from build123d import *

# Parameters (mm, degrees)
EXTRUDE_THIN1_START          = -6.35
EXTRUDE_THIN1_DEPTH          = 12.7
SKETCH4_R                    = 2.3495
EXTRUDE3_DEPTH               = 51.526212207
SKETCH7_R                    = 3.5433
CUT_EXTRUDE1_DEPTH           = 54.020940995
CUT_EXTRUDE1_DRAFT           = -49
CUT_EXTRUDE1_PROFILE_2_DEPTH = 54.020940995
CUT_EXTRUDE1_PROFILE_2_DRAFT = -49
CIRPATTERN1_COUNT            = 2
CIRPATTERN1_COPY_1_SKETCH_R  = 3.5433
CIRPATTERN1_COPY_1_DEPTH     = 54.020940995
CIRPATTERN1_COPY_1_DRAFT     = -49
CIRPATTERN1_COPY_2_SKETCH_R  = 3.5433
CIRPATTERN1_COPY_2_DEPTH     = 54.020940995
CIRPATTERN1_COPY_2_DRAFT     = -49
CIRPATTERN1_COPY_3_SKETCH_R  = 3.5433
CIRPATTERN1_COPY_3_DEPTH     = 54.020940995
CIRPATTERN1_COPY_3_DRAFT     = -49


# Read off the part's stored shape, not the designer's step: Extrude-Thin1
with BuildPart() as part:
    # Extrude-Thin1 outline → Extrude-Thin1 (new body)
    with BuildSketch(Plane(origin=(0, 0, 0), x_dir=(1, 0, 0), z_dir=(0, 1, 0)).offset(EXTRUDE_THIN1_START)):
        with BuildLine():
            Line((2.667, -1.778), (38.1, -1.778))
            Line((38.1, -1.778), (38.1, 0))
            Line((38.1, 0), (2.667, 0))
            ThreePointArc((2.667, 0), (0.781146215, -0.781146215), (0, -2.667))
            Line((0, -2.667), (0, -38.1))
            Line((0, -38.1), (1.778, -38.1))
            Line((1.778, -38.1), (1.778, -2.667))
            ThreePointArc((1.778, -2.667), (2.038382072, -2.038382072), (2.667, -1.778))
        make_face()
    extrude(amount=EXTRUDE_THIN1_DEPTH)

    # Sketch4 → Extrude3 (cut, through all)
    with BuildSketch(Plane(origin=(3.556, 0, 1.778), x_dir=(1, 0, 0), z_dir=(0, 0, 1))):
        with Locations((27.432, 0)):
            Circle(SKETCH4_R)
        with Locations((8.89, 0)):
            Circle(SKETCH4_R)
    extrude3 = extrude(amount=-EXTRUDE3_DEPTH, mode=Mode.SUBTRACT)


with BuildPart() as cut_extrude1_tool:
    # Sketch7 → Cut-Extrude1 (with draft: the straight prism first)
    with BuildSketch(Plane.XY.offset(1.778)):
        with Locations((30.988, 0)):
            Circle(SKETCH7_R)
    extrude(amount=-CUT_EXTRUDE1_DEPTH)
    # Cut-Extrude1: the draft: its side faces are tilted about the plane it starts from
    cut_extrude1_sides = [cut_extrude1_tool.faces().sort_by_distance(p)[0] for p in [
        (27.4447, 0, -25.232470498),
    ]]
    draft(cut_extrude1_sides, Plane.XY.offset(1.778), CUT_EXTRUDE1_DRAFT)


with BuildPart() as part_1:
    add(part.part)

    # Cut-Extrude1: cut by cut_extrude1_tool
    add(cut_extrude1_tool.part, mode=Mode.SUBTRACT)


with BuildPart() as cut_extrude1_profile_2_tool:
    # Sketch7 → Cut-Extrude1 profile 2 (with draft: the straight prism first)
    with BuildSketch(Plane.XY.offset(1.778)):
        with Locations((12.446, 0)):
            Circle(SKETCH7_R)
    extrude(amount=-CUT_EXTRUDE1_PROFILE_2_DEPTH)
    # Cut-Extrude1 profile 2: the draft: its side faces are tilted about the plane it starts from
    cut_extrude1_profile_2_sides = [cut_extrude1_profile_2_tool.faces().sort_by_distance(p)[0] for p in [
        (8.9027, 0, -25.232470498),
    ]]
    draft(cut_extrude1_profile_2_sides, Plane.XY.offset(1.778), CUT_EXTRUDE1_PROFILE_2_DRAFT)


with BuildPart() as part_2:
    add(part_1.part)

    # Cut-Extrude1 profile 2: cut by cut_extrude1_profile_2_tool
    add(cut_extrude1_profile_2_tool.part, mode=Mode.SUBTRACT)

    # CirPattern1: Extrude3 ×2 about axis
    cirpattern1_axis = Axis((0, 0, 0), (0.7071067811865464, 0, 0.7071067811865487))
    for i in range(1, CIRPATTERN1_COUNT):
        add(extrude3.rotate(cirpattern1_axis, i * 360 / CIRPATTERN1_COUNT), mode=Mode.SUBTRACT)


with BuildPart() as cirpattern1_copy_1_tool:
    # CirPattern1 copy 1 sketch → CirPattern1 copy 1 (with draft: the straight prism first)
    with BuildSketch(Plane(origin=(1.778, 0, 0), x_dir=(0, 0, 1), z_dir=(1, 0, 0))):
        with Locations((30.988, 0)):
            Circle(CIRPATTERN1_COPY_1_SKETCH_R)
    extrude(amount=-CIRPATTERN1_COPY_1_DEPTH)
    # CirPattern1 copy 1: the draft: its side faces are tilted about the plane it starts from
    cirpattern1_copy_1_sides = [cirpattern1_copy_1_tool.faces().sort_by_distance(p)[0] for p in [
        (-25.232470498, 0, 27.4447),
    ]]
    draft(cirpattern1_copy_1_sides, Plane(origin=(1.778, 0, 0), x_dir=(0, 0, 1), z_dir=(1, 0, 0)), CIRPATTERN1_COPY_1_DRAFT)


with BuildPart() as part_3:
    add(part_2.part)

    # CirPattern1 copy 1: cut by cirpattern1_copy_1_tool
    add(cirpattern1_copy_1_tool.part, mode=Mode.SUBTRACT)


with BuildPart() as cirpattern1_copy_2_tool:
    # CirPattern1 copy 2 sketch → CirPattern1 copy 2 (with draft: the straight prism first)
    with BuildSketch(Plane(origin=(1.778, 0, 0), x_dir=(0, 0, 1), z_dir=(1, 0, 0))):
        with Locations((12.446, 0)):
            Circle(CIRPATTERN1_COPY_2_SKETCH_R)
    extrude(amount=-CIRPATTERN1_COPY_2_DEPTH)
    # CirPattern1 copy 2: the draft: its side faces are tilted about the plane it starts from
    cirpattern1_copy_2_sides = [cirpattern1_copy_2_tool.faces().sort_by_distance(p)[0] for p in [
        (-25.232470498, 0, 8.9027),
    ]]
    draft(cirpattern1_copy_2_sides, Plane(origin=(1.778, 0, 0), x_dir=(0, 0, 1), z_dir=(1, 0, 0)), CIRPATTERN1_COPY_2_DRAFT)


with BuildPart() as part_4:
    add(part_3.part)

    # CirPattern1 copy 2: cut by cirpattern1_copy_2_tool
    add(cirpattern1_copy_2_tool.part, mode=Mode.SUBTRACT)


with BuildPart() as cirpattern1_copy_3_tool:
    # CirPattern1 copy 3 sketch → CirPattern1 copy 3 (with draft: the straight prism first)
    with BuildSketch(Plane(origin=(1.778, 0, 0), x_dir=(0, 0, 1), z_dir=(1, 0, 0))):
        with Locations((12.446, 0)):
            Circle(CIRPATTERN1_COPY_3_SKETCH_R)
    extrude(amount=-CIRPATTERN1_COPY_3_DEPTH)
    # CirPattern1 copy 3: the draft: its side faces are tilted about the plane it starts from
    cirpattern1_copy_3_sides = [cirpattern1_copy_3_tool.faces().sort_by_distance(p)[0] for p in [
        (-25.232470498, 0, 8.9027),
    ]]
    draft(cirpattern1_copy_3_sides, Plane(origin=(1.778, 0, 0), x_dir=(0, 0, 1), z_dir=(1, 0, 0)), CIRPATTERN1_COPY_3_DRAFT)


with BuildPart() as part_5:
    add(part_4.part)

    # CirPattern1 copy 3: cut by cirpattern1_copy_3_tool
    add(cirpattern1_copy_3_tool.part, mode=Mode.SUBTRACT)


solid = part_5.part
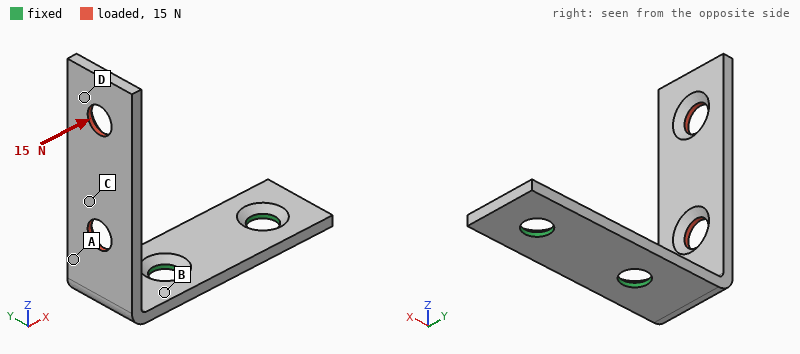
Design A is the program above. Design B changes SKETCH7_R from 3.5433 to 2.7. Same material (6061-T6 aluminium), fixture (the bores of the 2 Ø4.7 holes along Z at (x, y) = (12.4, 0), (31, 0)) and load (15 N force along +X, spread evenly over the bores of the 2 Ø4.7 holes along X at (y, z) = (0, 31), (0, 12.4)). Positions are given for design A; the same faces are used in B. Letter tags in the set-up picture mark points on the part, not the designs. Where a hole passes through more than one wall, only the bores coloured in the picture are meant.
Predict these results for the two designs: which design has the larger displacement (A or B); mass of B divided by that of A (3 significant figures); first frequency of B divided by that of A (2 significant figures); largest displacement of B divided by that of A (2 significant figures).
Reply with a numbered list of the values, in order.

1. A
2. 1.01
3. 1.1
4. 0.90
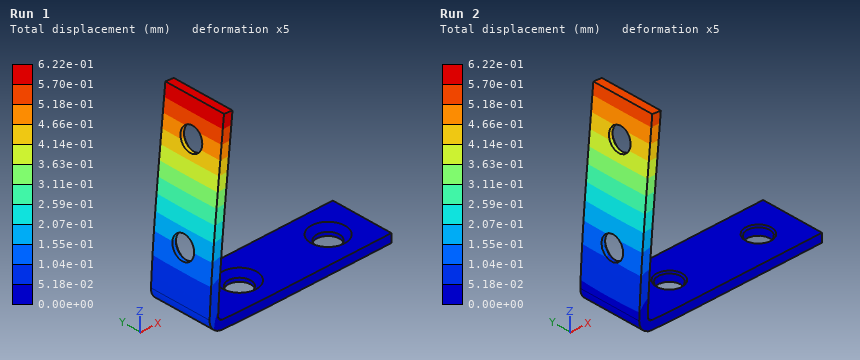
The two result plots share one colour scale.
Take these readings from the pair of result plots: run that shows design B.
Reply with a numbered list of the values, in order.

1. Run 2
